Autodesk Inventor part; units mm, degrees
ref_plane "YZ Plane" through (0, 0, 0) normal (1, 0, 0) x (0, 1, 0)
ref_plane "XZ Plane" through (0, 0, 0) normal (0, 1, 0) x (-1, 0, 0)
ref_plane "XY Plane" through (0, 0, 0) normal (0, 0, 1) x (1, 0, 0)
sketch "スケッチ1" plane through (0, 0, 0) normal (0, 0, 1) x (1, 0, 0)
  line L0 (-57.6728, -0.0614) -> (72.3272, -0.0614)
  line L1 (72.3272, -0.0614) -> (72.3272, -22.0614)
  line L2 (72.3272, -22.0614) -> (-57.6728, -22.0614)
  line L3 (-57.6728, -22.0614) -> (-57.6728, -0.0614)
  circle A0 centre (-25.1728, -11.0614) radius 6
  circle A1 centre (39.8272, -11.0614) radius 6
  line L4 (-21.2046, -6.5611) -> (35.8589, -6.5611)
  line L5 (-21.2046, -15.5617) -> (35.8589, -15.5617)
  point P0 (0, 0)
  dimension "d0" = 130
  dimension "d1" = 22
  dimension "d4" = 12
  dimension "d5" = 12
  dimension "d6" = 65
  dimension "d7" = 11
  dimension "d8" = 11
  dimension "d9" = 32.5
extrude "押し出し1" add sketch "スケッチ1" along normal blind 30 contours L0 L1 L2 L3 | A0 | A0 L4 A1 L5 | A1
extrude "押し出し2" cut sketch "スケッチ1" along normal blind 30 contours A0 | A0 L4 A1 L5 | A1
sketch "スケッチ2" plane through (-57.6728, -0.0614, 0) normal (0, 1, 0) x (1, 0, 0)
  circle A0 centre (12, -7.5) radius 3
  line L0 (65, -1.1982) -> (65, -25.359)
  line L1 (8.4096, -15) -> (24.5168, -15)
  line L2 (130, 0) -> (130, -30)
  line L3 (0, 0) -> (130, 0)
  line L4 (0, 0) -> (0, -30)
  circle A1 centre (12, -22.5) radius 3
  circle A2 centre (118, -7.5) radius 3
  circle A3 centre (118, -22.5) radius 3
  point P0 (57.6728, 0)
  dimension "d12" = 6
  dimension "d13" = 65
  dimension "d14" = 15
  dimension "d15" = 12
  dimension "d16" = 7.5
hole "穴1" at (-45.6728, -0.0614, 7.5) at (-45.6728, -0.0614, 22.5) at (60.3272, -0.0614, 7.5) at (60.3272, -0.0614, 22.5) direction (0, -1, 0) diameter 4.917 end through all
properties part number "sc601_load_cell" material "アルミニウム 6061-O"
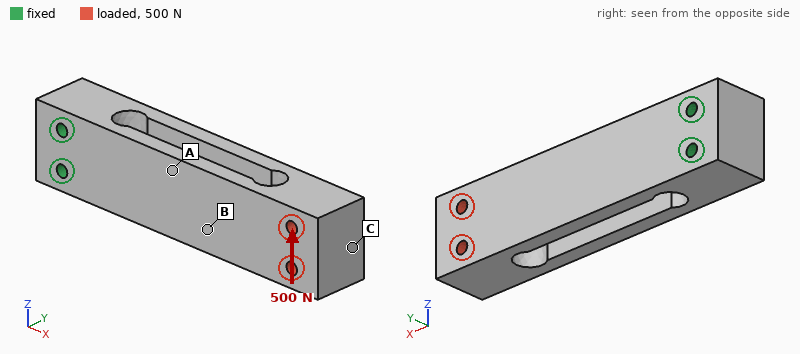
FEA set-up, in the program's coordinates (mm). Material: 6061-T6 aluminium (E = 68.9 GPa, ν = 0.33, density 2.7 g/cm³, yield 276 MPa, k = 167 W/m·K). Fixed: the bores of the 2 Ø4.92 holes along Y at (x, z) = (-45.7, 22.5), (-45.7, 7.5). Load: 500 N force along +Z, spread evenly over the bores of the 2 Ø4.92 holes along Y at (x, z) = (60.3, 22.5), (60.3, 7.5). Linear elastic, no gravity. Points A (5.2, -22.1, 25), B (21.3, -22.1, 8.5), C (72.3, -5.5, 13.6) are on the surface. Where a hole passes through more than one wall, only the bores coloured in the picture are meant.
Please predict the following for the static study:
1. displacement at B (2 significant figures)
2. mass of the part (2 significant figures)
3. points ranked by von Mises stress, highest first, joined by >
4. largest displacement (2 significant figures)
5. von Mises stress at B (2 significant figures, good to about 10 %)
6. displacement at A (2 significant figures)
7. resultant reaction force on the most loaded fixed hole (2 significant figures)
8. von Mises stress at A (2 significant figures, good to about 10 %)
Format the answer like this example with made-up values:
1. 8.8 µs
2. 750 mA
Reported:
1. 0.049 mm
2. 170 g
3. A > B > C
4. 0.12 mm
5. 5.4 MPa
6. 0.031 mm
7. 3.0 kN
8. 9.8 MPa
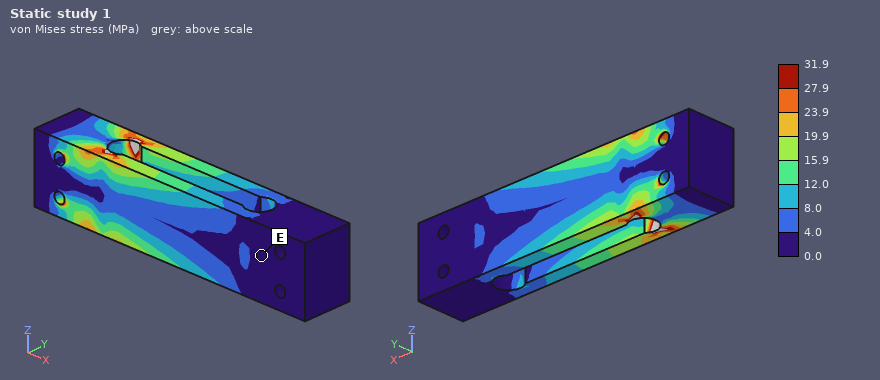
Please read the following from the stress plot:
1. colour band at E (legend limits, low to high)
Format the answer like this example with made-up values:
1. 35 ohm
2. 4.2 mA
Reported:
1. 0.0 to 4.0 MPa
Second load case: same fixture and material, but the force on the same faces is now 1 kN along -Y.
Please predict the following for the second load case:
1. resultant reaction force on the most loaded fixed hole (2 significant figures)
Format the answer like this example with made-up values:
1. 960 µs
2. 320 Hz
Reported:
1. 500 N
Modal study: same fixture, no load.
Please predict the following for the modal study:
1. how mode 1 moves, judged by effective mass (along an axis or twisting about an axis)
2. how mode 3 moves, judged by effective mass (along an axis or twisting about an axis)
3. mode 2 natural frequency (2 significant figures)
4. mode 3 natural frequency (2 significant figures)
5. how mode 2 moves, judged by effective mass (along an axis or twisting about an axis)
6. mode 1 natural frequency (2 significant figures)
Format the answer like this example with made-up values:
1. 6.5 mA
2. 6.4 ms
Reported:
1. along Y
2. twisting about X
3. 1400 Hz
4. 2900 Hz
5. along Z
6. 680 Hz
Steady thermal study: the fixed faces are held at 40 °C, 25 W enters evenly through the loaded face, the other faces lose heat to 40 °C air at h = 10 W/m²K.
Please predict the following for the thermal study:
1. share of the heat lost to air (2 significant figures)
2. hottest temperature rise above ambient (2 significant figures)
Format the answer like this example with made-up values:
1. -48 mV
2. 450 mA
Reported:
1. 12 %
2. 35 K
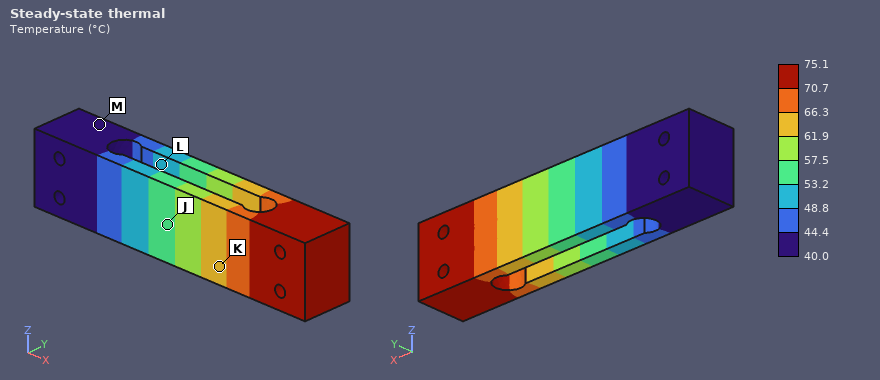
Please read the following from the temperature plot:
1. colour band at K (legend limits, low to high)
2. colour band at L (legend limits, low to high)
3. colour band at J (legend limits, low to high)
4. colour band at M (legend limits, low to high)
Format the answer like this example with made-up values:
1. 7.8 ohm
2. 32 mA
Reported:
1. 61.9 to 66.3 °C
2. 48.8 to 53.2 °C
3. 53.2 to 57.5 °C
4. 40.0 to 44.4 °C
